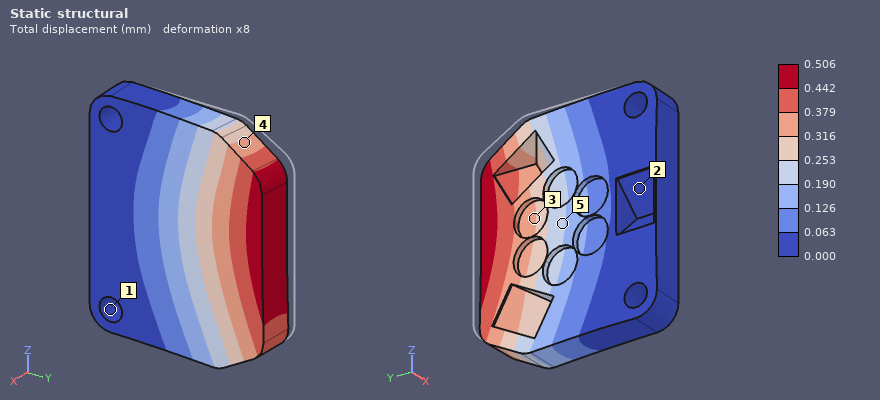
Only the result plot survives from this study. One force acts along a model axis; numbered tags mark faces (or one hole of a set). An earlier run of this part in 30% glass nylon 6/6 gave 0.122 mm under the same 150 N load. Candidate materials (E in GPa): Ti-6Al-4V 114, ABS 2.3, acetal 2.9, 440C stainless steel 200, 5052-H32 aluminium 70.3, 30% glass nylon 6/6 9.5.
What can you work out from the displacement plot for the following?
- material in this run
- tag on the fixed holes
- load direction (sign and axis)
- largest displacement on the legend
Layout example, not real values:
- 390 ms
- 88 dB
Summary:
- ABS
- 1
- +X
- 0.506 mm
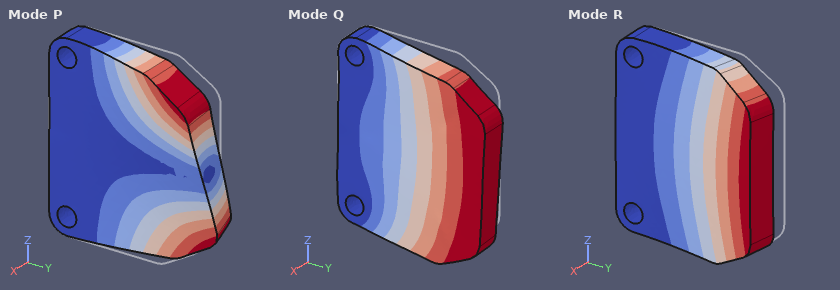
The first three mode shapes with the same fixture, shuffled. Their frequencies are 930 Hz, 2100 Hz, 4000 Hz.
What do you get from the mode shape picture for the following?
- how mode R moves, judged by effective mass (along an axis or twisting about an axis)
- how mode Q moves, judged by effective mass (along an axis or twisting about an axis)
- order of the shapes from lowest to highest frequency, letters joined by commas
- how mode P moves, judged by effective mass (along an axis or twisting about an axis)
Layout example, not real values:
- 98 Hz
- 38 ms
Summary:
- along X
- along Z
- R, P, Q
- twisting about Y
